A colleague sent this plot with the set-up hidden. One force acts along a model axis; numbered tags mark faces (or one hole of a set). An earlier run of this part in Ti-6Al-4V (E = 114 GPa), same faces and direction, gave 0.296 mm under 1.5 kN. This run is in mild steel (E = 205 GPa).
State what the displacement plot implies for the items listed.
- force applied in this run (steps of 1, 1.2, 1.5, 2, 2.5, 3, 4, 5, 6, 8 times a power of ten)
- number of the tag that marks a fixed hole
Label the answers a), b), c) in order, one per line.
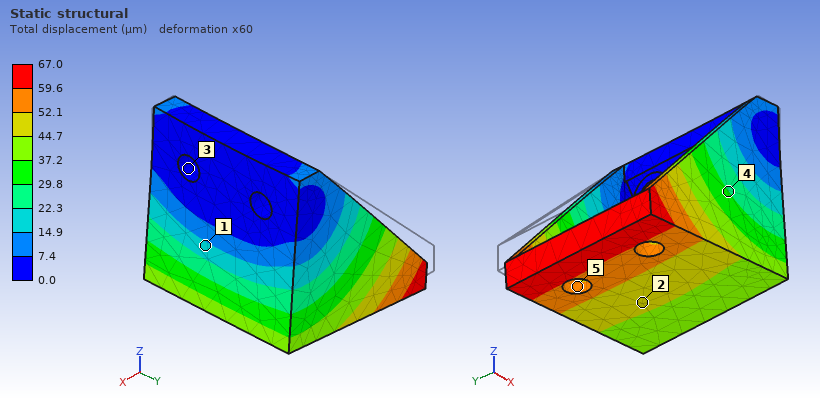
a) 600 N
b) 3
